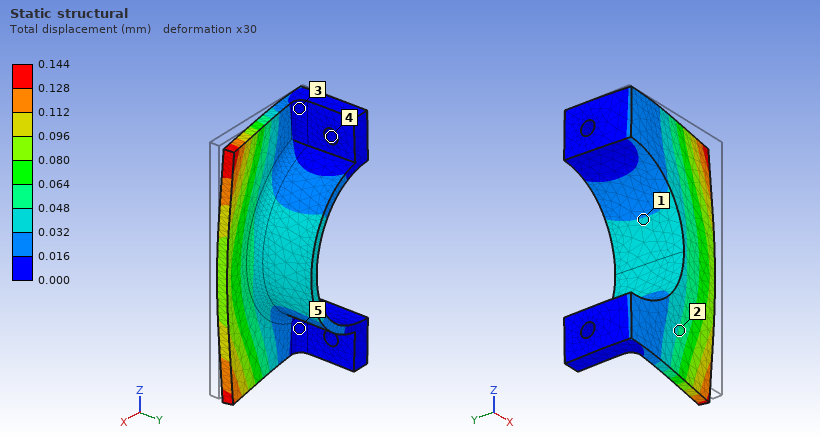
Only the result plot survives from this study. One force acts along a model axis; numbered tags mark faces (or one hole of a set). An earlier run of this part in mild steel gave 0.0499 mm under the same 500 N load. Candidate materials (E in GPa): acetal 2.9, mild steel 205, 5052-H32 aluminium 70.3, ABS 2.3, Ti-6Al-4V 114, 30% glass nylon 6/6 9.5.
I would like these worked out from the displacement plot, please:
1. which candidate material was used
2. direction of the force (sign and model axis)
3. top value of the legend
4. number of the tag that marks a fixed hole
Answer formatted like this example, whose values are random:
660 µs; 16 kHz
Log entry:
5052-H32 aluminium; +Y; 0.144 mm; 4
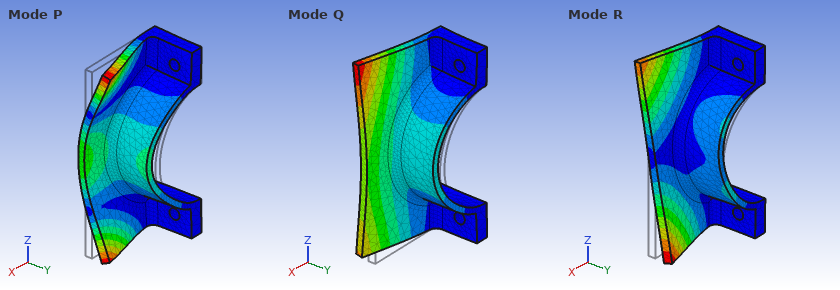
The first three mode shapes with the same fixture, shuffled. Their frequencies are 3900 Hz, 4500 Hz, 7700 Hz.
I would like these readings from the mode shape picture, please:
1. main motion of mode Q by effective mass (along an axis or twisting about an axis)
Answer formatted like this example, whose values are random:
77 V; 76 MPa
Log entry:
along Y
